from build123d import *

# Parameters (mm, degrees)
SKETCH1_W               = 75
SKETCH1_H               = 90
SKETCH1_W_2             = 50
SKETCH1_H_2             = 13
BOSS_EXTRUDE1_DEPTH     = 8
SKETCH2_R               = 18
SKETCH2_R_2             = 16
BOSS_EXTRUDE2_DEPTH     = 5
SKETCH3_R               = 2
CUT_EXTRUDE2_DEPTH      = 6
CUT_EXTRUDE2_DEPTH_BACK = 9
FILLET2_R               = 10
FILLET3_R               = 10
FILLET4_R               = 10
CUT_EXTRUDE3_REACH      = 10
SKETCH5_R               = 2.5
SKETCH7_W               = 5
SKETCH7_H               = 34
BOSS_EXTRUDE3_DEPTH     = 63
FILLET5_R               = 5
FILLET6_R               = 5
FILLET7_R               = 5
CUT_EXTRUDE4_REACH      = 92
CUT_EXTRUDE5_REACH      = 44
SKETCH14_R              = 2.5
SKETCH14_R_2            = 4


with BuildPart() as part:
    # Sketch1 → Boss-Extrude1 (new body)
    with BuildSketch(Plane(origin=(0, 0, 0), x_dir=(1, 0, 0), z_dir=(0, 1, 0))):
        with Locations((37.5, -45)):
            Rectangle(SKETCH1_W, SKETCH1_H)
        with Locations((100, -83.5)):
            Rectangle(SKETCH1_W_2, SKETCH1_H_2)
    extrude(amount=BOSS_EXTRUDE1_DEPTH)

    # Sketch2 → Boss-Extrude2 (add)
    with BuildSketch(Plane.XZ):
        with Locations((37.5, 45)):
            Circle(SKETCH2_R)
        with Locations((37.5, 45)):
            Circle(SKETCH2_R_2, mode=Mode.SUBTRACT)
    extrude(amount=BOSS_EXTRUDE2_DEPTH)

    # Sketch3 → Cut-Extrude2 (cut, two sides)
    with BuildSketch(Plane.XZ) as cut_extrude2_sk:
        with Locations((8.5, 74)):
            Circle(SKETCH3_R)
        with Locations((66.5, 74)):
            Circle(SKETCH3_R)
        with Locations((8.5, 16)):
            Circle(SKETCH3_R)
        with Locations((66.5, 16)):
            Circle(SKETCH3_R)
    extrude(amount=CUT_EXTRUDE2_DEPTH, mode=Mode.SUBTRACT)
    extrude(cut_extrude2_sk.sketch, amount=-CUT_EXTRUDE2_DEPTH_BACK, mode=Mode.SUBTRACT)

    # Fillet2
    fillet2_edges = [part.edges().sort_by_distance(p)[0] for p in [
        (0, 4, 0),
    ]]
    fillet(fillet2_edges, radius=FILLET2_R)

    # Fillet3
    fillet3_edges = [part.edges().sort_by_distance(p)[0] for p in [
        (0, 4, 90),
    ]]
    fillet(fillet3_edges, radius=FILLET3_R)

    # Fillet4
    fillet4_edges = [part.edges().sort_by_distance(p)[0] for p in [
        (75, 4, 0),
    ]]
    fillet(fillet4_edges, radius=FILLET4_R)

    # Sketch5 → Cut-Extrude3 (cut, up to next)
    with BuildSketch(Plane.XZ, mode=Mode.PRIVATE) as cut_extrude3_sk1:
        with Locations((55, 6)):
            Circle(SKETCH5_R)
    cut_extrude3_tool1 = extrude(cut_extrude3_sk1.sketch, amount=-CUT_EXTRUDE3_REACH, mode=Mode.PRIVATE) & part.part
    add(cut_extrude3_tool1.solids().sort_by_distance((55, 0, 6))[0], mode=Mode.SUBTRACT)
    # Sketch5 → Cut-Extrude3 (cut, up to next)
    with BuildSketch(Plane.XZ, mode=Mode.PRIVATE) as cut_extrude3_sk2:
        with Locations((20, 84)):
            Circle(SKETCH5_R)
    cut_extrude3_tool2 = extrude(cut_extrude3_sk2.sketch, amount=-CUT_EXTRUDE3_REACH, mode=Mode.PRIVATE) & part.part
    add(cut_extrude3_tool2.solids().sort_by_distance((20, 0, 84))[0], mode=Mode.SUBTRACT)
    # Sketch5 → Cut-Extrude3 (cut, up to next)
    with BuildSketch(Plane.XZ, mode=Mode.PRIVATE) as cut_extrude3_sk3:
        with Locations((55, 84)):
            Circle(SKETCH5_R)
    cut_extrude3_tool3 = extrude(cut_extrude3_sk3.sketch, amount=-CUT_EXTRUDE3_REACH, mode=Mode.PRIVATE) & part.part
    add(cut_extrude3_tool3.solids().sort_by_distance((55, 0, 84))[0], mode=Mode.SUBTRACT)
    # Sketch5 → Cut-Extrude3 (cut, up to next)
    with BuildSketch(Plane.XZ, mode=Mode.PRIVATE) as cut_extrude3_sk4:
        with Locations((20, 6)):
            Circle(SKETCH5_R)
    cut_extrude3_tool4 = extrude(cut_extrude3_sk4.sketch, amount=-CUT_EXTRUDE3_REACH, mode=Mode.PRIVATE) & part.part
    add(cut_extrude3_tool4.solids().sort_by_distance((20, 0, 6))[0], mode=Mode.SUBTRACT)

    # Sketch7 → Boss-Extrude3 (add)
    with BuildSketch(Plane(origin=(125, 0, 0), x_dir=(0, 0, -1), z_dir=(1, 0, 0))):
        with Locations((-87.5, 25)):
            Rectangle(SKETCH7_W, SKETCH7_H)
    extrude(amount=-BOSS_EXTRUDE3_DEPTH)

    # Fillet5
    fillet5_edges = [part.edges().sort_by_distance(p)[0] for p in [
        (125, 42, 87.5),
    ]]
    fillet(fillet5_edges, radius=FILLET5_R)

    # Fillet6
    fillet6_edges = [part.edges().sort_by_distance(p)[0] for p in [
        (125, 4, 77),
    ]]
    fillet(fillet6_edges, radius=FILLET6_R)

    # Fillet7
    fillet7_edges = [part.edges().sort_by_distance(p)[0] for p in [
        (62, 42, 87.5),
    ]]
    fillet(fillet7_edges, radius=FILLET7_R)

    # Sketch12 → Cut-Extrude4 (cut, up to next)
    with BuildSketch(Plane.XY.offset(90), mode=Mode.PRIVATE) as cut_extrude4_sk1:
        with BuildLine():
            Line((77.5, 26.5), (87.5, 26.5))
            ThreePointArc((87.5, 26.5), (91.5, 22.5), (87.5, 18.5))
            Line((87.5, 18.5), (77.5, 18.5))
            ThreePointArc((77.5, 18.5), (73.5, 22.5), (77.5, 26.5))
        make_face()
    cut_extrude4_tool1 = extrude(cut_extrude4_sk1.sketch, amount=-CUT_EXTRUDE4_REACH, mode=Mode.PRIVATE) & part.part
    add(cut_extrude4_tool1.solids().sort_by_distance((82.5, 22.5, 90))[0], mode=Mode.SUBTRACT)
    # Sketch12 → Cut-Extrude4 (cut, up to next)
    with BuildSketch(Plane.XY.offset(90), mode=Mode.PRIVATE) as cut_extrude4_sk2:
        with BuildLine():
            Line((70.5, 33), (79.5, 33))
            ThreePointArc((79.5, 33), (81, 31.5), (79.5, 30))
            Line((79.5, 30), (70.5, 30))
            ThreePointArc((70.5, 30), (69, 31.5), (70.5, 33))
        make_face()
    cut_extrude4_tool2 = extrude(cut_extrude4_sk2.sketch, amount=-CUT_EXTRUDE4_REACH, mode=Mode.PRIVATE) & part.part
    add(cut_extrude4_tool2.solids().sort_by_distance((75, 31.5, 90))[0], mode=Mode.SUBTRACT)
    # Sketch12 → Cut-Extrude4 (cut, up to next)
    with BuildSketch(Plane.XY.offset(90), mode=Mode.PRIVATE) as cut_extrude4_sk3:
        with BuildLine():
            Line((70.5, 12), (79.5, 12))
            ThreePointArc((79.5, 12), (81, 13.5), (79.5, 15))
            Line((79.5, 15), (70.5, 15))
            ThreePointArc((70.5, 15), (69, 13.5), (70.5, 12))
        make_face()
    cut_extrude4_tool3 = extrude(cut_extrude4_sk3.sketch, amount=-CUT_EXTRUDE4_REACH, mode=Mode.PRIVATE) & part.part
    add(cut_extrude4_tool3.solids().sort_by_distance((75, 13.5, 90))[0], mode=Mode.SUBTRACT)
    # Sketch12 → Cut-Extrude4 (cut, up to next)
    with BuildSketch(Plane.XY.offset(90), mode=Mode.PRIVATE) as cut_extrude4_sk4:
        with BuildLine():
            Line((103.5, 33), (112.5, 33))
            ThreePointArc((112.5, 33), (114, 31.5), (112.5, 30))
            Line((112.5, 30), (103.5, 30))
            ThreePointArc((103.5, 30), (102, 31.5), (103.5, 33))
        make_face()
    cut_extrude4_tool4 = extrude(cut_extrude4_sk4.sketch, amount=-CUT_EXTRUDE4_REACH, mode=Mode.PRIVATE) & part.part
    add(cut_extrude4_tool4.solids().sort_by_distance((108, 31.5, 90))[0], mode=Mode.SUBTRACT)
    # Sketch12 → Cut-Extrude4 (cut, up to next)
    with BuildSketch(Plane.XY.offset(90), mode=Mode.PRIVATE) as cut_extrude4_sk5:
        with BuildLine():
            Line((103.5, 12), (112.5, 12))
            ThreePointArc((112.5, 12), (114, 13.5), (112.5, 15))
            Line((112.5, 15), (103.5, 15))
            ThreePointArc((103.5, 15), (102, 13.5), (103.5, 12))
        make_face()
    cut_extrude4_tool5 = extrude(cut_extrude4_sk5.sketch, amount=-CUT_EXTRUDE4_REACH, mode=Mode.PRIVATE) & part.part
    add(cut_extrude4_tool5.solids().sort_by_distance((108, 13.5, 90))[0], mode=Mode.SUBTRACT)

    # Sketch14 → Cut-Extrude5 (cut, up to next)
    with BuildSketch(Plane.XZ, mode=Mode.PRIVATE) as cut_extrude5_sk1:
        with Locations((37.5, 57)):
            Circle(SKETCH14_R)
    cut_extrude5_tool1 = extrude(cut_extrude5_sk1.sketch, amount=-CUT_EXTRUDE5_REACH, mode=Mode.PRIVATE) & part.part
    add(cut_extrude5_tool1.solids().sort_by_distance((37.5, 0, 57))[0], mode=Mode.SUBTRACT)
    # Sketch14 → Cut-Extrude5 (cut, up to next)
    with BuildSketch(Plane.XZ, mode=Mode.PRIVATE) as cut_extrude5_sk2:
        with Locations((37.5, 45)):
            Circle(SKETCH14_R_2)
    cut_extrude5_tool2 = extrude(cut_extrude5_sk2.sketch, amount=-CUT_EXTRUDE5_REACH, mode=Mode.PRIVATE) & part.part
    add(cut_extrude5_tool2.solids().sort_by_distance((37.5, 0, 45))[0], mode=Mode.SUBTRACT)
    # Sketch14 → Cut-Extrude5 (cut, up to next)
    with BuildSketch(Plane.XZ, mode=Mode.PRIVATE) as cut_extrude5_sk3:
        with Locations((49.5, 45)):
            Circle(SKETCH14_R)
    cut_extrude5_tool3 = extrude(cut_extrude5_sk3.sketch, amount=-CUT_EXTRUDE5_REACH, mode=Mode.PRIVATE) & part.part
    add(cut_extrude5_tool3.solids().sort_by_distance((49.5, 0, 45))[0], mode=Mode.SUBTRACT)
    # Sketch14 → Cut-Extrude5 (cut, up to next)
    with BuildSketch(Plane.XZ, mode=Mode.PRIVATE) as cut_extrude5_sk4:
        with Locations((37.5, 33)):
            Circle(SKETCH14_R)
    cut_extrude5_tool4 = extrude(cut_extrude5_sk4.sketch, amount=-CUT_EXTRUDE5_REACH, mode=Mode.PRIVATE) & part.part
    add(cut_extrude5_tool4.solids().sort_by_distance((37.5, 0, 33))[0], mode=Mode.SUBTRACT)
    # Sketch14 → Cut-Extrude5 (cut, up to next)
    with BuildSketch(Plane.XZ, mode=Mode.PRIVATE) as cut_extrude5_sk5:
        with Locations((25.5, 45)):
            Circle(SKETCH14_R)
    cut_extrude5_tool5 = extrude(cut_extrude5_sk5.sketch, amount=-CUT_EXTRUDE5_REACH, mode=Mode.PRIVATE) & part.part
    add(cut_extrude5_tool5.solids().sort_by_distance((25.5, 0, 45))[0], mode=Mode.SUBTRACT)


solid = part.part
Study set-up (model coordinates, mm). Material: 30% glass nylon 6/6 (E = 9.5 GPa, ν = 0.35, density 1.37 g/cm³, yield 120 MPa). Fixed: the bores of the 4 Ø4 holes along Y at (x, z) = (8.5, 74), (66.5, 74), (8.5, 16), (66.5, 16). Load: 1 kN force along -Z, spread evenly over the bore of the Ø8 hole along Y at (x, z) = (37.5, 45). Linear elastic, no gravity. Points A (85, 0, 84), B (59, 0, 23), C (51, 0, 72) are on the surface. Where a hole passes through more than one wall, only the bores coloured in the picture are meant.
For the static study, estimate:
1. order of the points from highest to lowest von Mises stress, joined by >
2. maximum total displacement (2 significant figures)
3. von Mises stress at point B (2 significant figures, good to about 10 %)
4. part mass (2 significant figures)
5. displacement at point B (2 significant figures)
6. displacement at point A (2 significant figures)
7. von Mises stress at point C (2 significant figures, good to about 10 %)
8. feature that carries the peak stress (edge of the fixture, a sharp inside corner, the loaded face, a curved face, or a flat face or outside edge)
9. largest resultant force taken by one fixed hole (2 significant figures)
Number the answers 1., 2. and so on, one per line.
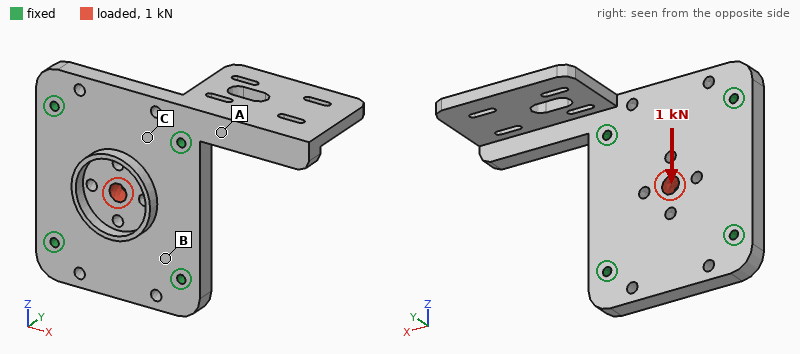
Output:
1. B > C > A
2. 13 µm
3. 2.1 MPa
4. 92 g
5. 2.8 µm
6. 2.0 µm
7. 1.1 MPa
8. the loaded face
9. 270 N
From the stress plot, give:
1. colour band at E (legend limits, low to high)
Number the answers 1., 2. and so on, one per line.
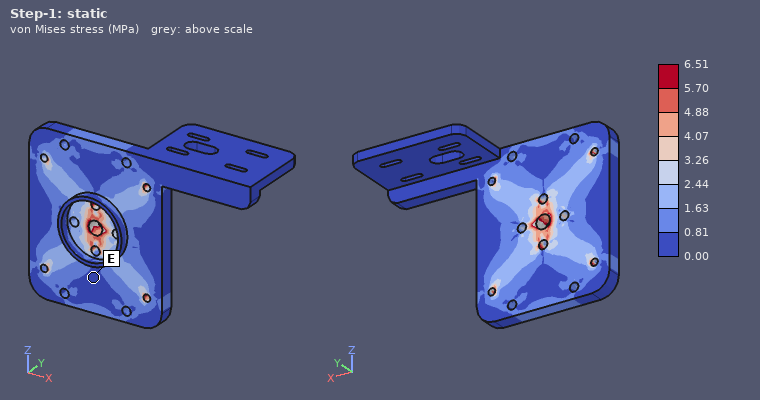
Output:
1. 0.00 to 0.81 MPa
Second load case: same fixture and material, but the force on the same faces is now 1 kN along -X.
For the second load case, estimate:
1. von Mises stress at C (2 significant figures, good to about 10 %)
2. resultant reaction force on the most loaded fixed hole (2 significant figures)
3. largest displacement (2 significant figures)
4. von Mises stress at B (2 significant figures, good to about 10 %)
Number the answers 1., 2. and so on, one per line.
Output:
1. 1.1 MPa
2. 280 N
3. 14 µm
4. 2.3 MPa
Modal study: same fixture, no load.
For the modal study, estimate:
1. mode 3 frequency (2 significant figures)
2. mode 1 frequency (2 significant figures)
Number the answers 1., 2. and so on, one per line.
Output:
1. 1400 Hz
2. 680 Hz
